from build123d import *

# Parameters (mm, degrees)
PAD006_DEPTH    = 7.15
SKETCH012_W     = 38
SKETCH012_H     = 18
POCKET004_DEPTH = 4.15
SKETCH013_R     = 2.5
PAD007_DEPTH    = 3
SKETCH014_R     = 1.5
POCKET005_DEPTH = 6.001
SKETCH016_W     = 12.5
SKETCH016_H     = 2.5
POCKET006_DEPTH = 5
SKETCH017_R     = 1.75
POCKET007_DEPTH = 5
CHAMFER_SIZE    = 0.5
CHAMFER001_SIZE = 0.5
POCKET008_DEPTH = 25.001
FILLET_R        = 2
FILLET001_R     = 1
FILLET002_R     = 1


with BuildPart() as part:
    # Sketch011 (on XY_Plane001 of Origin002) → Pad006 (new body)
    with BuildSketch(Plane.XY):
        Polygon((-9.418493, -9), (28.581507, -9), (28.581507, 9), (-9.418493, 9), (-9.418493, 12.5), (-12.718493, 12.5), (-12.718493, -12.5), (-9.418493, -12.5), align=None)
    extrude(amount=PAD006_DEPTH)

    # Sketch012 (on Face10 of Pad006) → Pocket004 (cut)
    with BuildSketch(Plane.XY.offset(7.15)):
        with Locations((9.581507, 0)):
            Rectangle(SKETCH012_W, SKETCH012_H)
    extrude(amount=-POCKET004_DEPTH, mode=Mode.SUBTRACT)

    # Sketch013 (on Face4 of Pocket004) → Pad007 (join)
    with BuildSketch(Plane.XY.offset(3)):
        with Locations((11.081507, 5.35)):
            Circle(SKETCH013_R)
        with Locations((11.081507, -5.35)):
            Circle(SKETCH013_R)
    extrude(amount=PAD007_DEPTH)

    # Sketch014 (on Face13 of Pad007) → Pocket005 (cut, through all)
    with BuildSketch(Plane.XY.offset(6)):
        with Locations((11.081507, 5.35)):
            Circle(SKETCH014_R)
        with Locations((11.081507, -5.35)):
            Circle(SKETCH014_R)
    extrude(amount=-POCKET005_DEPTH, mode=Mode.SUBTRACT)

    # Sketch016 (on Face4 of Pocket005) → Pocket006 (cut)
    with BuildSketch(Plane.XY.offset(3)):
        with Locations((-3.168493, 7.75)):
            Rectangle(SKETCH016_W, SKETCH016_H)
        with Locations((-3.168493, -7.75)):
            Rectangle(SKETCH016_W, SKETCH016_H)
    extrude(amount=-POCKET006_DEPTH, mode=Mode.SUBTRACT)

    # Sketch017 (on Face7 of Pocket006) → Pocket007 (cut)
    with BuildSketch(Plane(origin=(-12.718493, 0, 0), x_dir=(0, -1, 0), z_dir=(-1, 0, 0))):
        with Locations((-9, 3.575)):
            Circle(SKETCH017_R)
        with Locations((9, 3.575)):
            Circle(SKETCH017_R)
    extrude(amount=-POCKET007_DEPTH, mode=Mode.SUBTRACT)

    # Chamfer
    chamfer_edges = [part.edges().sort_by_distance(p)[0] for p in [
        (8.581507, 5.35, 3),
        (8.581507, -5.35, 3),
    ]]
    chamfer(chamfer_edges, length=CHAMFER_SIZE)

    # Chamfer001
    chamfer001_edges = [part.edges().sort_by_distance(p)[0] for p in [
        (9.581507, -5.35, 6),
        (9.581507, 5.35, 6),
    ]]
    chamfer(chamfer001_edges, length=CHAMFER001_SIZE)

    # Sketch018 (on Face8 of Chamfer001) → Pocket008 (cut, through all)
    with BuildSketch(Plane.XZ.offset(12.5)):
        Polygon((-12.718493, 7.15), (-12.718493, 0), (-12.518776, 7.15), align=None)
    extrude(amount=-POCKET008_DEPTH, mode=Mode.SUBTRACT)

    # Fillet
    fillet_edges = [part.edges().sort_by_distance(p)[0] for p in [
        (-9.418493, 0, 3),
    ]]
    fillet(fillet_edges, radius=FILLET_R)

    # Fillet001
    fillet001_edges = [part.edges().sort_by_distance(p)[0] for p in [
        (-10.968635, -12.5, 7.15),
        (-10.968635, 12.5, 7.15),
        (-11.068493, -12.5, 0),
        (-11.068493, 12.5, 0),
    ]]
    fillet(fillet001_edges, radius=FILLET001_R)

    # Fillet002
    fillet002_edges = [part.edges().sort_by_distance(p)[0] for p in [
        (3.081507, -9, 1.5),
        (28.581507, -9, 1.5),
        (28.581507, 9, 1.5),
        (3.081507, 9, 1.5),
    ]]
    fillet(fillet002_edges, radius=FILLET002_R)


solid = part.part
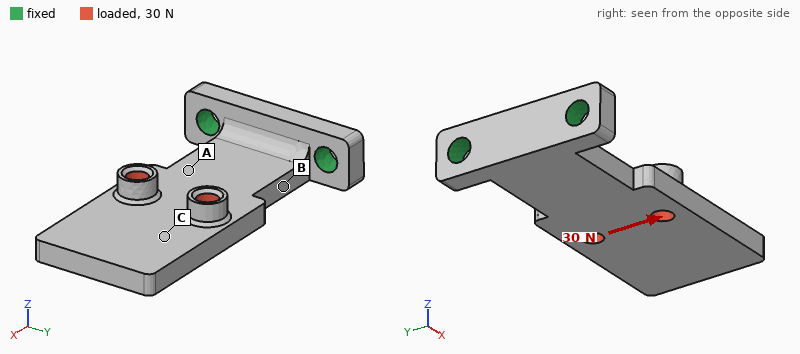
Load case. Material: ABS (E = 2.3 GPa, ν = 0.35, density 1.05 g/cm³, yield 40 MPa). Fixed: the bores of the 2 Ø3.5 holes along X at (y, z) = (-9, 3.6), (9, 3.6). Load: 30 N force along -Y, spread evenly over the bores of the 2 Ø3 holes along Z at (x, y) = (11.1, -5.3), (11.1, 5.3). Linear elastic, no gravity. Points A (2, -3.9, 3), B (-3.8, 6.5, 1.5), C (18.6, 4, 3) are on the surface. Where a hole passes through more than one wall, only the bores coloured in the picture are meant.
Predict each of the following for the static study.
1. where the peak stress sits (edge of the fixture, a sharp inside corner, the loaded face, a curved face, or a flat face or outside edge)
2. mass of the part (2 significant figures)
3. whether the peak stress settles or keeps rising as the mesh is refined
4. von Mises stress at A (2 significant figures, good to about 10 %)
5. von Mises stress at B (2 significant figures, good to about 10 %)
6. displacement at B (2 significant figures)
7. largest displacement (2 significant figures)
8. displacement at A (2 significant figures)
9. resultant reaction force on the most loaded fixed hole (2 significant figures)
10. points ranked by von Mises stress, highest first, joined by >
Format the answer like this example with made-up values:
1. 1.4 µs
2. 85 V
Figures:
1. a sharp inside corner
2. 2.5 g
3. keeps rising
4. 3.8 MPa
5. 5.5 MPa
6. 0.049 mm
7. 0.29 mm
8. 0.081 mm
9. 50 N
10. B > A > C
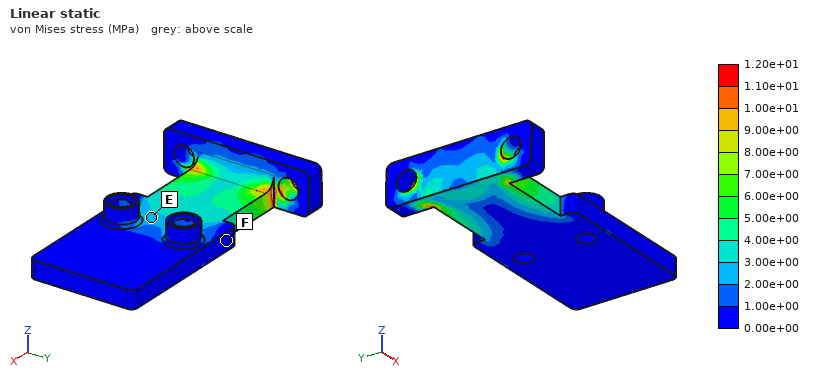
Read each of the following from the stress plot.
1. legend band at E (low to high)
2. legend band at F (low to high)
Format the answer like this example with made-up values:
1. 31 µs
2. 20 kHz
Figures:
1. 2.00e+00 to 3.00e+00 MPa
2. 0.00e+00 to 1.00e+00 MPa
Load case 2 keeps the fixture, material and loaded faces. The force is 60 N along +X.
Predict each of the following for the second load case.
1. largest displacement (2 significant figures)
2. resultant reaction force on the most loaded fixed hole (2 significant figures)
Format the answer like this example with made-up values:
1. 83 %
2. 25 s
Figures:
1. 0.55 mm
2. 32 N
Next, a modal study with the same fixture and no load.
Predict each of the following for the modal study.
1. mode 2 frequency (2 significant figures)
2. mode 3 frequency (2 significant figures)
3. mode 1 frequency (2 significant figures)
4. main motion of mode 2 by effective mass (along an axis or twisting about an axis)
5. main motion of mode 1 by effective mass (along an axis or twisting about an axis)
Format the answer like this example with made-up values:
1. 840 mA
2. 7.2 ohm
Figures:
1. 1400 Hz
2. 1800 Hz
3. 390 Hz
4. along Y
5. along Z
